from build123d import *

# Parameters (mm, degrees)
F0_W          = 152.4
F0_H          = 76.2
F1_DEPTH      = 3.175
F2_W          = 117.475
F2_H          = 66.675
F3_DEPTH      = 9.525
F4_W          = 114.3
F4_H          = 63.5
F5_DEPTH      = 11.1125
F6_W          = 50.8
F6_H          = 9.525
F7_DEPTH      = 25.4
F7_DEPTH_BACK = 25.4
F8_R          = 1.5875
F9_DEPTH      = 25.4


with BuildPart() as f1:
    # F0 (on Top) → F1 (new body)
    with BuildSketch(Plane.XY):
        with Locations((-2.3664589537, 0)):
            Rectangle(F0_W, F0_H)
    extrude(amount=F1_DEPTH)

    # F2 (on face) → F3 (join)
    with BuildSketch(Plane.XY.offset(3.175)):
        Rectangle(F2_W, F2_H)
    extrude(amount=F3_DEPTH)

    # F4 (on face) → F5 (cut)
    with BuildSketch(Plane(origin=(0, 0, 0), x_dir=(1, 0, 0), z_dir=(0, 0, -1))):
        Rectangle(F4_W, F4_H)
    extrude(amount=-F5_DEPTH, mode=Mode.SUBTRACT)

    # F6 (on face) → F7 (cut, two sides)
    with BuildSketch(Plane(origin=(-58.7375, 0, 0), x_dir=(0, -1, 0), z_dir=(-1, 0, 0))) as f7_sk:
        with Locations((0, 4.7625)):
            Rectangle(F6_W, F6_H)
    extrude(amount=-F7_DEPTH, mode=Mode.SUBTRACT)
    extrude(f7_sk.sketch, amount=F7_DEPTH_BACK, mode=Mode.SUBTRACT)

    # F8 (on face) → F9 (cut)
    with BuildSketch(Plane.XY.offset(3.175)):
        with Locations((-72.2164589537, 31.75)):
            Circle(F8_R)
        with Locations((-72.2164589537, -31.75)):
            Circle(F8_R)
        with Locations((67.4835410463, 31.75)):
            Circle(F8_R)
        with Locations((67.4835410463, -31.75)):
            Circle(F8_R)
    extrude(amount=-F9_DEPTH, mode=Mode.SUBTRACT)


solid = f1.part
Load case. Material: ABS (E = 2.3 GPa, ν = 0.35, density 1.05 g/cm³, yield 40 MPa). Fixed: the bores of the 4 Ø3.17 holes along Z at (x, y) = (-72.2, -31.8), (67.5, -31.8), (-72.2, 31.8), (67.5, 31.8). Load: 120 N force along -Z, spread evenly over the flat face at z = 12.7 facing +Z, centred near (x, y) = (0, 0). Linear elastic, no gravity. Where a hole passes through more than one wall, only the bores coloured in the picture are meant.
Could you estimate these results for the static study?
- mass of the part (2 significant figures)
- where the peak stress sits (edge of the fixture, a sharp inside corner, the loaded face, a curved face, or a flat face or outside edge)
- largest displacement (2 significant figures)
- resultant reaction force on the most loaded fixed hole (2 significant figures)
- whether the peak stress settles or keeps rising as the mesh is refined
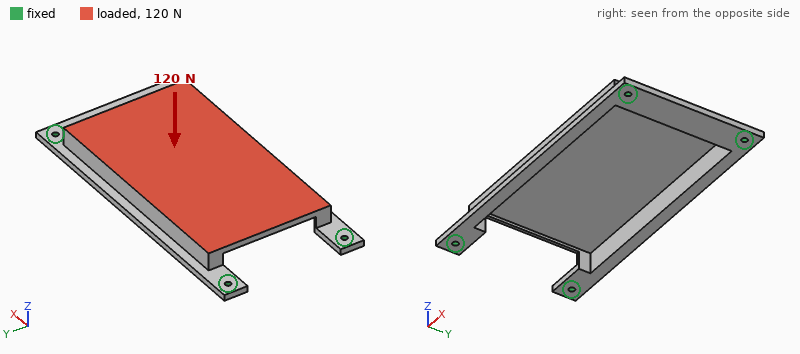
28 g
edge of the fixture
1.8 mm
63 N
keeps rising
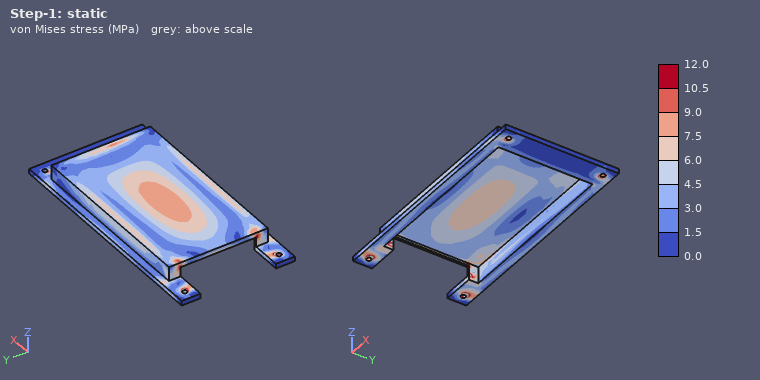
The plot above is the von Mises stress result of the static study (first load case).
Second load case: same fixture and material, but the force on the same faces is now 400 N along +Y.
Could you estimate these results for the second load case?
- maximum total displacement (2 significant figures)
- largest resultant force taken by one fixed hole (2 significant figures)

0.59 mm
230 N
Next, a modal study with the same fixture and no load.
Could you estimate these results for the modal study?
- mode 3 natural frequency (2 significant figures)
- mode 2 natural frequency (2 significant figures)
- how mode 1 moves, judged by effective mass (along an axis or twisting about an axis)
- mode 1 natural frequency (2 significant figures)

730 Hz
660 Hz
along Z
430 Hz
